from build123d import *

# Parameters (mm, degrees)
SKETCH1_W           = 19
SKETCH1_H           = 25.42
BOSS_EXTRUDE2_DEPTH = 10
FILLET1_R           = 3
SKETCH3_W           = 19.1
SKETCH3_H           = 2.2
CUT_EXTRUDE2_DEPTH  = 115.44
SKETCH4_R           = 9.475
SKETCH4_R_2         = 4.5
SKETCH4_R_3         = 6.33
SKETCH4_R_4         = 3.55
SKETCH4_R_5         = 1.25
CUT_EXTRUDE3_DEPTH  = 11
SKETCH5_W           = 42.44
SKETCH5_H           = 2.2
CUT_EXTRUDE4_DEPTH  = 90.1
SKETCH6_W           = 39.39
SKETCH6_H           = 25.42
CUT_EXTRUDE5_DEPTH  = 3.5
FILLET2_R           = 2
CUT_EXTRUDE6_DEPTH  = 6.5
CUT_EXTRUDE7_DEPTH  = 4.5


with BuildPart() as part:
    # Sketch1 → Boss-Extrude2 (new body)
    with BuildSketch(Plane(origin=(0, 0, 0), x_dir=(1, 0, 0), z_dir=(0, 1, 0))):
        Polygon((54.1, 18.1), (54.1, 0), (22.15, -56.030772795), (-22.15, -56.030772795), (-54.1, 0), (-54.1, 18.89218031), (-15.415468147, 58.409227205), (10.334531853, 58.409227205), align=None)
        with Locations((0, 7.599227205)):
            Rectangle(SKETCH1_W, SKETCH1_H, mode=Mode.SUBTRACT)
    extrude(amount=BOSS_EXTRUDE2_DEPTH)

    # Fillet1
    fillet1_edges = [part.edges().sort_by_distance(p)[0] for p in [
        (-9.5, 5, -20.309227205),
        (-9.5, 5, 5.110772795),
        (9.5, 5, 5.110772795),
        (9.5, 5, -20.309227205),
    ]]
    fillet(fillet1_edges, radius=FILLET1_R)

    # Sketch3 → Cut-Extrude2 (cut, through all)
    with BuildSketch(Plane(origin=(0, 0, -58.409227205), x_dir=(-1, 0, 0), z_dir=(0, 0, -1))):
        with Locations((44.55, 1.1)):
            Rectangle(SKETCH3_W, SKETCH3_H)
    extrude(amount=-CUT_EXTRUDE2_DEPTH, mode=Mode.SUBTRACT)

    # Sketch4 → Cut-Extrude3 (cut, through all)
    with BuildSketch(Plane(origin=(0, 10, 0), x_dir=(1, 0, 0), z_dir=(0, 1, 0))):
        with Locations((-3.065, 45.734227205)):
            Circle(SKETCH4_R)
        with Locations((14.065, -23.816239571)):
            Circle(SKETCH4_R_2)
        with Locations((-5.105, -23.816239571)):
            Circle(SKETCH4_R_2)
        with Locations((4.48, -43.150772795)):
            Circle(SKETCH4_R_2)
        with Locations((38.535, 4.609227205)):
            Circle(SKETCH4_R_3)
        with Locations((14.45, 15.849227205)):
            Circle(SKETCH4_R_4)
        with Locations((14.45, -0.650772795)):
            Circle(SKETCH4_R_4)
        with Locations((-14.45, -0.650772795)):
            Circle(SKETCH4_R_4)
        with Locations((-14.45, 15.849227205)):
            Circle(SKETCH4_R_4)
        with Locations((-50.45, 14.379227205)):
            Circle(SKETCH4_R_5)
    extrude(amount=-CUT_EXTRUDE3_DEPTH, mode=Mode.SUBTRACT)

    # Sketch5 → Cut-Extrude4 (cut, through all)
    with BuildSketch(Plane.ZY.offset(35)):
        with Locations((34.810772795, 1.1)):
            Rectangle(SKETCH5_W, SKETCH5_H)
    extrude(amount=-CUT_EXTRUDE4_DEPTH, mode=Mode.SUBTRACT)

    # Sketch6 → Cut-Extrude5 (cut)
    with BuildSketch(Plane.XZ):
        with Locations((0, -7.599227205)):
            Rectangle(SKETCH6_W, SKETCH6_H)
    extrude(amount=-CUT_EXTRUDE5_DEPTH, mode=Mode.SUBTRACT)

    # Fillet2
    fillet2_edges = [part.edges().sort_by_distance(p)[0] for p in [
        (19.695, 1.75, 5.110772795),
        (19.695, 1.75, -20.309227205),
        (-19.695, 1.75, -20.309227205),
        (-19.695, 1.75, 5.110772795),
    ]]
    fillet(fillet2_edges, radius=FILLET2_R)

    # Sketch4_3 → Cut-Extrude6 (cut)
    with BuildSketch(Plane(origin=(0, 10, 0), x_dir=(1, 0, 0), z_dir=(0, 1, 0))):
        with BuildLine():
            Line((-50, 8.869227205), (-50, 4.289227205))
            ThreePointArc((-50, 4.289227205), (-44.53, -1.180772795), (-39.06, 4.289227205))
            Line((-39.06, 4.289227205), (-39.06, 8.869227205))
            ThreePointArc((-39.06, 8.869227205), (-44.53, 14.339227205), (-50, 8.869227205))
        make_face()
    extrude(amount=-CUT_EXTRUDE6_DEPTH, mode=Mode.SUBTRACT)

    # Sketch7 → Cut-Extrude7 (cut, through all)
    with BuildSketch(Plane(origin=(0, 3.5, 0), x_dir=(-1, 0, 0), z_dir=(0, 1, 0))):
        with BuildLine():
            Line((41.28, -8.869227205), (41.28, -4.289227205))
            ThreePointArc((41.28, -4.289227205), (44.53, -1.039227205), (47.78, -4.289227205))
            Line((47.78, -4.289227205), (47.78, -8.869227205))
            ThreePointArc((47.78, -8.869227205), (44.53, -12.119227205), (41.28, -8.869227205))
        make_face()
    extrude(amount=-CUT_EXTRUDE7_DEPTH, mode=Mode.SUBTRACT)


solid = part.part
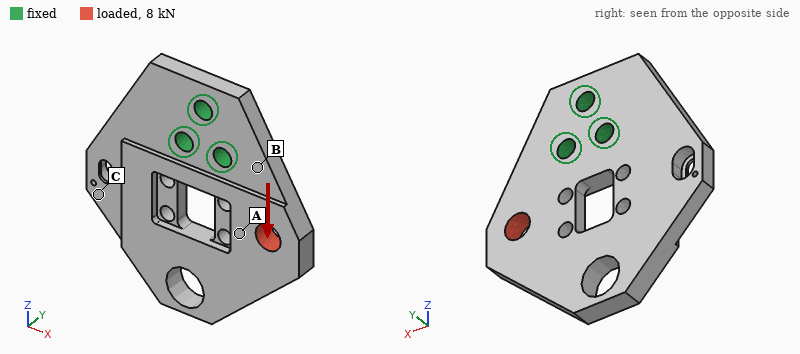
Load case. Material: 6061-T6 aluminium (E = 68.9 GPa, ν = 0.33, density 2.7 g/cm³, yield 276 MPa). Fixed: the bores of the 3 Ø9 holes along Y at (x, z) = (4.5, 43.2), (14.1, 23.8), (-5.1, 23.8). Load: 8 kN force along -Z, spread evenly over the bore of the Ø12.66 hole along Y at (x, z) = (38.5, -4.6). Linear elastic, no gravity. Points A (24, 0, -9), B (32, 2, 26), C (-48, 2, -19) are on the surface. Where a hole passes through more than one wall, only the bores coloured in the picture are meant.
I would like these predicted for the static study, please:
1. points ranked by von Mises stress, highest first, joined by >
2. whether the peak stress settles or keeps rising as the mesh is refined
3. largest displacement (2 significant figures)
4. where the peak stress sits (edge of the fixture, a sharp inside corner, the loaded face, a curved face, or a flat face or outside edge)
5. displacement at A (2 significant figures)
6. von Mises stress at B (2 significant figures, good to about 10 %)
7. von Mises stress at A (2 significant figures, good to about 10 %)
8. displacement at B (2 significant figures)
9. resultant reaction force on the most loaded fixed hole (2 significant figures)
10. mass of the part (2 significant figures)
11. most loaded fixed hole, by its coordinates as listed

B > A > C
keeps rising
0.10 mm
edge of the fixture
0.051 mm
54 MPa
20 MPa
0.024 mm
9.5 kN
180 g
(14.1, 23.8)
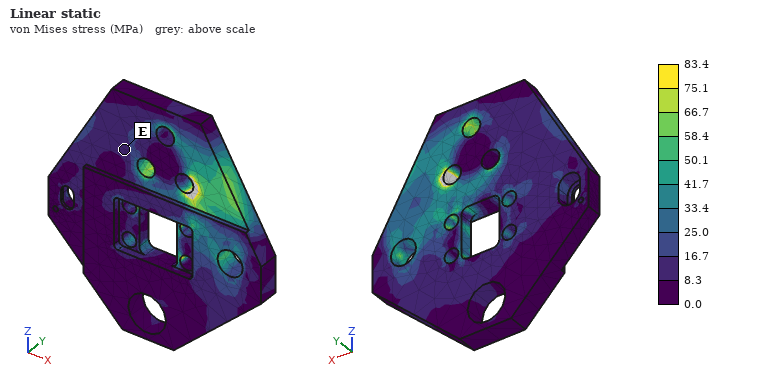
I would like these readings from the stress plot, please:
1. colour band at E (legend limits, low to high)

8.3 to 16.7 MPa
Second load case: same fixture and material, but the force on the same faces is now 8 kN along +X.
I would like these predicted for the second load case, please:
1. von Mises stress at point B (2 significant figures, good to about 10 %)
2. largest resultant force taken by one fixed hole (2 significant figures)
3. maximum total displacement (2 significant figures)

25 MPa
7.6 kN
100 µm
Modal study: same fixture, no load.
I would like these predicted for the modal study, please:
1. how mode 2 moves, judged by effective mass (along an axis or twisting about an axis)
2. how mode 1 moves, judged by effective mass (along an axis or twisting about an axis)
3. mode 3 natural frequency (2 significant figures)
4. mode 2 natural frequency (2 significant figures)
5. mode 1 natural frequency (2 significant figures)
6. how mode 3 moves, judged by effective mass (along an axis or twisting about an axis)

twisting about Z
along Y
3800 Hz
2000 Hz
1100 Hz
along X
